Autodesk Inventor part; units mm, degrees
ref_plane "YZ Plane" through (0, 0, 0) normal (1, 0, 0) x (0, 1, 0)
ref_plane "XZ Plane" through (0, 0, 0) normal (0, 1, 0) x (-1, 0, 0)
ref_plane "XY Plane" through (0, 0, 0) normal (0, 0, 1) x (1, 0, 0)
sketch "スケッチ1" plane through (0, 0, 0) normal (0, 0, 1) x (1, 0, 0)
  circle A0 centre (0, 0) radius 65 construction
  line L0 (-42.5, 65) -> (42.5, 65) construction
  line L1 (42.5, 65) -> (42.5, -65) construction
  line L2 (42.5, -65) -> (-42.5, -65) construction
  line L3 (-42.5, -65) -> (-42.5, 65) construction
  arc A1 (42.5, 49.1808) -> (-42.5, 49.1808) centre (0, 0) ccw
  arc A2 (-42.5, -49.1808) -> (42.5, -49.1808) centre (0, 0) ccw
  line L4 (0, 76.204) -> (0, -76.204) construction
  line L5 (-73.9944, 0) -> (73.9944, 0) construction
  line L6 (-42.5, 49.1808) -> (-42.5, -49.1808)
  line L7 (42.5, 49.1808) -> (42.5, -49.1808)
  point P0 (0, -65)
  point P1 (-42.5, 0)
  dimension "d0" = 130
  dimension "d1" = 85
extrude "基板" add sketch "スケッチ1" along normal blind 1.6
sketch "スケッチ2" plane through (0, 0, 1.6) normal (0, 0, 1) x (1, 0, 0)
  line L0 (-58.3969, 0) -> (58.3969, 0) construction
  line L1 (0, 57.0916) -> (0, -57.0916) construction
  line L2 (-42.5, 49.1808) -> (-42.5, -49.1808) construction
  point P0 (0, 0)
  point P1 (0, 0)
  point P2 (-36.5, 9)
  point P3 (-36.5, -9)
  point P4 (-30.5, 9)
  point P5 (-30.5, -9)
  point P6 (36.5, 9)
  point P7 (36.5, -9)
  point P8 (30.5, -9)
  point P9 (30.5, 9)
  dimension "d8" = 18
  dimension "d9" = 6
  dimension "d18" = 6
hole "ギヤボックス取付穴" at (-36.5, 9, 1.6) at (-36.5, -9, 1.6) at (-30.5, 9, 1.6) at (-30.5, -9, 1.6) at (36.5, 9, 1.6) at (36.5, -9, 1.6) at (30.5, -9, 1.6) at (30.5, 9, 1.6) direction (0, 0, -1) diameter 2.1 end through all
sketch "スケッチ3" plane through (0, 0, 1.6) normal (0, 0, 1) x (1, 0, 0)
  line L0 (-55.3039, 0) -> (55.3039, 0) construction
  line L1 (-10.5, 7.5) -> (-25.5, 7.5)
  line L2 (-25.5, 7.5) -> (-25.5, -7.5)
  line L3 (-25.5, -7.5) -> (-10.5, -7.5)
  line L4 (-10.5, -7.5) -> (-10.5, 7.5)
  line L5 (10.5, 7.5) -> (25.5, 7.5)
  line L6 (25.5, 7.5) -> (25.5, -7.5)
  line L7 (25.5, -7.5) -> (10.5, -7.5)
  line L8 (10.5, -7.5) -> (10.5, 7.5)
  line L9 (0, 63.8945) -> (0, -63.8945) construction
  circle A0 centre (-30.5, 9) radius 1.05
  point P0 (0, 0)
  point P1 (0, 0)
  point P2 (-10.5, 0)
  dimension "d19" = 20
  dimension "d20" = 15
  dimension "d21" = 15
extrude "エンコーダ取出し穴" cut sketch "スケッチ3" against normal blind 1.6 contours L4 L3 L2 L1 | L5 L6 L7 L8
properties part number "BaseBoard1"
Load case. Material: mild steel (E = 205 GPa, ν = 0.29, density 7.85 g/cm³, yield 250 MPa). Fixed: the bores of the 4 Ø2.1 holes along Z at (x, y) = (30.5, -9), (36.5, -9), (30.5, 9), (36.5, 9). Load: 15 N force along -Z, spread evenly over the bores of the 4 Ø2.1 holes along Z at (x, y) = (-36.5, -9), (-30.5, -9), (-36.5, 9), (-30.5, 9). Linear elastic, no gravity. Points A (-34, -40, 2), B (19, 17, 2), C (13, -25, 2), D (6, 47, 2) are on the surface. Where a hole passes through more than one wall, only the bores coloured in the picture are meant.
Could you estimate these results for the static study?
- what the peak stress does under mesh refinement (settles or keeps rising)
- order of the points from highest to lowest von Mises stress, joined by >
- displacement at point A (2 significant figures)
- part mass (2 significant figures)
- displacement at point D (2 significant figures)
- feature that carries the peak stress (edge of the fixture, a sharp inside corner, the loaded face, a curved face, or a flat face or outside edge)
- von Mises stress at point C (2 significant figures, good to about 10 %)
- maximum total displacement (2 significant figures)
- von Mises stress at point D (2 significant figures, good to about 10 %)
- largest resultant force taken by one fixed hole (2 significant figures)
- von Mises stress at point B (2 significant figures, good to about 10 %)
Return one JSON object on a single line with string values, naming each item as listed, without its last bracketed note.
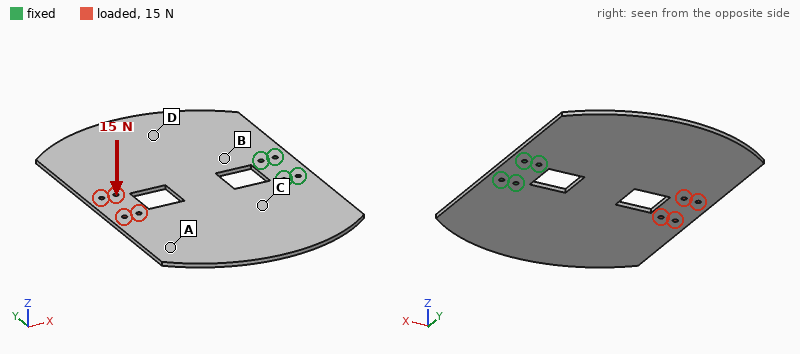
{"what the peak stress does under mesh refinement": "keeps rising", "order of the points from highest to lowest von Mises stress, joined by >": "B > C > D > A", "displacement at point A": "0.29 mm", "part mass": "120 g", "displacement at point D": "0.083 mm", "feature that carries the peak stress": "edge of the fixture", "von Mises stress at point C": "18 MPa", "maximum total displacement": "0.37 mm", "von Mises stress at point D": "9.6 MPa", "largest resultant force taken by one fixed hole": "47 N", "von Mises stress at point B": "27 MPa"}
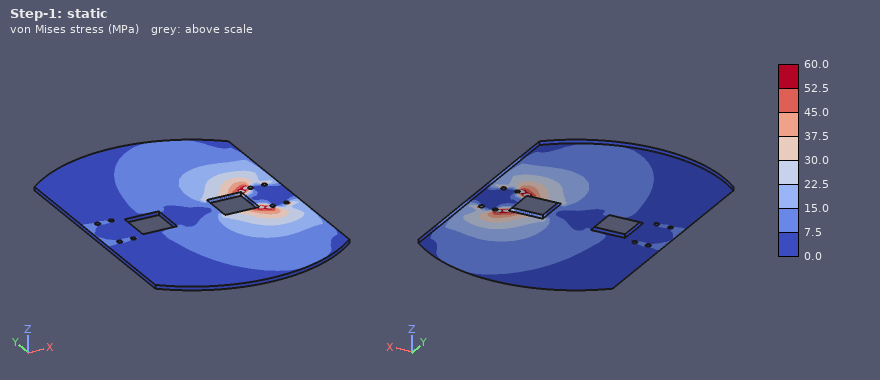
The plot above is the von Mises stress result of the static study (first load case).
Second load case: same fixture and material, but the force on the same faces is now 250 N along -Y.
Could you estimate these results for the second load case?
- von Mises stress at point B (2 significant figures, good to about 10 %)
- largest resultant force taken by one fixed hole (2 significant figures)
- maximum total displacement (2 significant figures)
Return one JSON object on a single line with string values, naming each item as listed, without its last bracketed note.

{"von Mises stress at point B": "13 MPa", "largest resultant force taken by one fixed hole": "560 N", "maximum total displacement": "35 µm"}
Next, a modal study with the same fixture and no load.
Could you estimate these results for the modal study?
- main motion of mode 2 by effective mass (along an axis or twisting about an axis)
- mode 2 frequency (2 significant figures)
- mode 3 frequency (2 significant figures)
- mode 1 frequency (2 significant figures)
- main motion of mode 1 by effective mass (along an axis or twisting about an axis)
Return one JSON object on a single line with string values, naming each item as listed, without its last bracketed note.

{"main motion of mode 2 by effective mass": "twisting about X", "mode 2 frequency": "230 Hz", "mode 3 frequency": "470 Hz", "mode 1 frequency": "170 Hz", "main motion of mode 1 by effective mass": "along Z"}
